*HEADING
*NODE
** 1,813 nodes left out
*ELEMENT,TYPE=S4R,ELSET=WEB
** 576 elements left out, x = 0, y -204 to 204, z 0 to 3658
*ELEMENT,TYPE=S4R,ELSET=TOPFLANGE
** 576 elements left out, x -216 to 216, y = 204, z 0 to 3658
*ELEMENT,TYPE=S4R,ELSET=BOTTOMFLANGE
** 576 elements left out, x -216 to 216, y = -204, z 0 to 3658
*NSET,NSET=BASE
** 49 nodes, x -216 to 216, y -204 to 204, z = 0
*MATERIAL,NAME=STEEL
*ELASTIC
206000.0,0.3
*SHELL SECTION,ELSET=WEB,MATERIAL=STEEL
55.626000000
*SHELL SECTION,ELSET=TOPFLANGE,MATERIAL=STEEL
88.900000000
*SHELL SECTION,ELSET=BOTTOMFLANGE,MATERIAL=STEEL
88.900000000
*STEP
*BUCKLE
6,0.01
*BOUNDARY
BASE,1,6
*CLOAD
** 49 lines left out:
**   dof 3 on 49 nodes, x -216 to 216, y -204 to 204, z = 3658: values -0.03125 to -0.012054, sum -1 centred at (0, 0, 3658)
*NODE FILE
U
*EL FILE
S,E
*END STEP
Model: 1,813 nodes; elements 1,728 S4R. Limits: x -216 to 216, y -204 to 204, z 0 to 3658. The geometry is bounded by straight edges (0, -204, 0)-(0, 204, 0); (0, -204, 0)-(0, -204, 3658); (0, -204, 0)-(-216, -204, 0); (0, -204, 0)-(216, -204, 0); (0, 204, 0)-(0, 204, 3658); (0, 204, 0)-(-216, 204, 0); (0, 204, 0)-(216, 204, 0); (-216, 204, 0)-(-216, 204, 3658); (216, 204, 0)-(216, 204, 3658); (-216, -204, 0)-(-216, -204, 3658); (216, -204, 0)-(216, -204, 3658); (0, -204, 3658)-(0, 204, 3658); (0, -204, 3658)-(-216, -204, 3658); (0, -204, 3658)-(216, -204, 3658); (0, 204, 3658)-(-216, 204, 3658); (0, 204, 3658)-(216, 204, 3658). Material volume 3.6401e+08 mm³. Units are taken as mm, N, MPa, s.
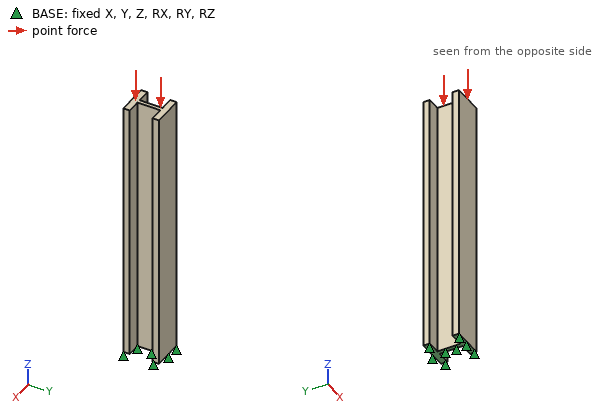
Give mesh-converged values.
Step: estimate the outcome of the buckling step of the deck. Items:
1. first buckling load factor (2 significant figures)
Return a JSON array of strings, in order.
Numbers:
["4.5e+07"]
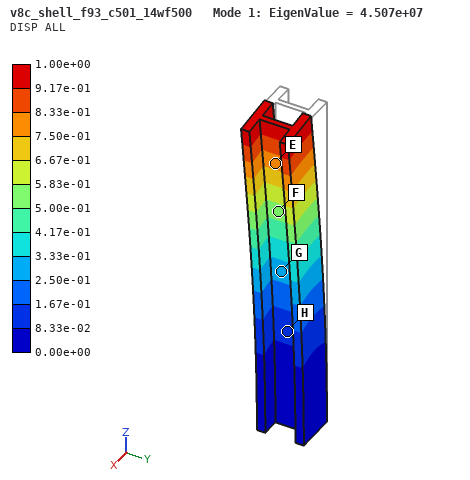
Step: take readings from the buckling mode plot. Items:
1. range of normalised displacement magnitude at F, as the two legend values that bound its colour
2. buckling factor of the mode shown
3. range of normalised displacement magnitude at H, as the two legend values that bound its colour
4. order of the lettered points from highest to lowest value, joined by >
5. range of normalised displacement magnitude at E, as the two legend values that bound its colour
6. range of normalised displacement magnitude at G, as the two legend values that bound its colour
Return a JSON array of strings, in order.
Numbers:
["5.00e-01 to 5.83e-01", "4.507e+07", "8.33e-02 to 1.67e-01", "E > F > G > H", "7.50e-01 to 8.33e-01", "2.50e-01 to 3.33e-01"]
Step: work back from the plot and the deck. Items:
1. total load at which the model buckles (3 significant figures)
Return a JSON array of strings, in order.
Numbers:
["4.51e+07 N"]
